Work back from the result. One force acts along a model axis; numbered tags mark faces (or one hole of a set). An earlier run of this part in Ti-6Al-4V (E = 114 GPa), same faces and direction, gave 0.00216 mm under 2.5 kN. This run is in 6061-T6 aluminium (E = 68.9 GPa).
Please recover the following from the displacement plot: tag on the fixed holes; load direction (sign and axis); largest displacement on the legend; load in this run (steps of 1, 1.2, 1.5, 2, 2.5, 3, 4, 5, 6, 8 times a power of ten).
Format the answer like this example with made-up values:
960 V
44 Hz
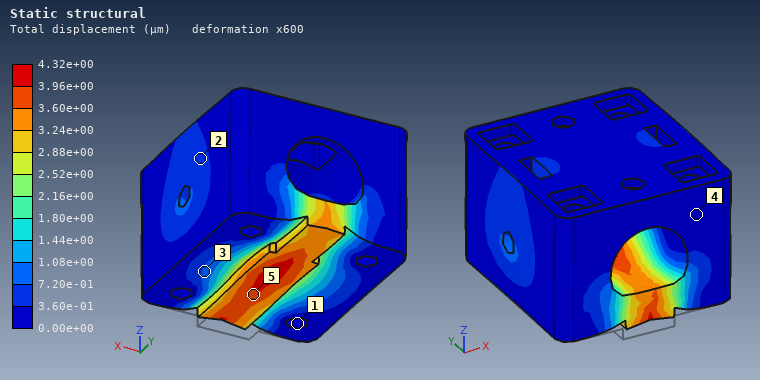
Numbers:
1
+Z
4.32e+00 µm
3 kN
